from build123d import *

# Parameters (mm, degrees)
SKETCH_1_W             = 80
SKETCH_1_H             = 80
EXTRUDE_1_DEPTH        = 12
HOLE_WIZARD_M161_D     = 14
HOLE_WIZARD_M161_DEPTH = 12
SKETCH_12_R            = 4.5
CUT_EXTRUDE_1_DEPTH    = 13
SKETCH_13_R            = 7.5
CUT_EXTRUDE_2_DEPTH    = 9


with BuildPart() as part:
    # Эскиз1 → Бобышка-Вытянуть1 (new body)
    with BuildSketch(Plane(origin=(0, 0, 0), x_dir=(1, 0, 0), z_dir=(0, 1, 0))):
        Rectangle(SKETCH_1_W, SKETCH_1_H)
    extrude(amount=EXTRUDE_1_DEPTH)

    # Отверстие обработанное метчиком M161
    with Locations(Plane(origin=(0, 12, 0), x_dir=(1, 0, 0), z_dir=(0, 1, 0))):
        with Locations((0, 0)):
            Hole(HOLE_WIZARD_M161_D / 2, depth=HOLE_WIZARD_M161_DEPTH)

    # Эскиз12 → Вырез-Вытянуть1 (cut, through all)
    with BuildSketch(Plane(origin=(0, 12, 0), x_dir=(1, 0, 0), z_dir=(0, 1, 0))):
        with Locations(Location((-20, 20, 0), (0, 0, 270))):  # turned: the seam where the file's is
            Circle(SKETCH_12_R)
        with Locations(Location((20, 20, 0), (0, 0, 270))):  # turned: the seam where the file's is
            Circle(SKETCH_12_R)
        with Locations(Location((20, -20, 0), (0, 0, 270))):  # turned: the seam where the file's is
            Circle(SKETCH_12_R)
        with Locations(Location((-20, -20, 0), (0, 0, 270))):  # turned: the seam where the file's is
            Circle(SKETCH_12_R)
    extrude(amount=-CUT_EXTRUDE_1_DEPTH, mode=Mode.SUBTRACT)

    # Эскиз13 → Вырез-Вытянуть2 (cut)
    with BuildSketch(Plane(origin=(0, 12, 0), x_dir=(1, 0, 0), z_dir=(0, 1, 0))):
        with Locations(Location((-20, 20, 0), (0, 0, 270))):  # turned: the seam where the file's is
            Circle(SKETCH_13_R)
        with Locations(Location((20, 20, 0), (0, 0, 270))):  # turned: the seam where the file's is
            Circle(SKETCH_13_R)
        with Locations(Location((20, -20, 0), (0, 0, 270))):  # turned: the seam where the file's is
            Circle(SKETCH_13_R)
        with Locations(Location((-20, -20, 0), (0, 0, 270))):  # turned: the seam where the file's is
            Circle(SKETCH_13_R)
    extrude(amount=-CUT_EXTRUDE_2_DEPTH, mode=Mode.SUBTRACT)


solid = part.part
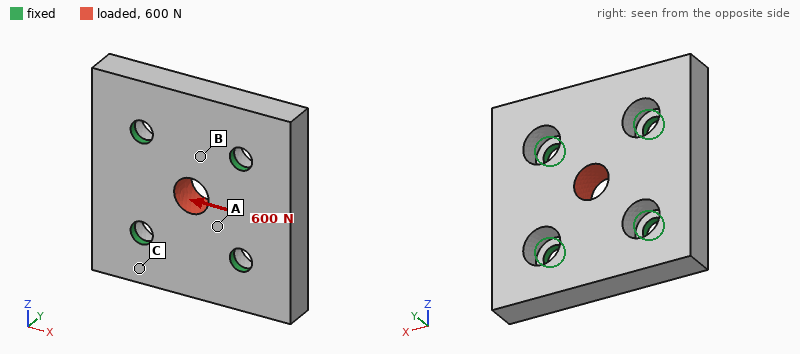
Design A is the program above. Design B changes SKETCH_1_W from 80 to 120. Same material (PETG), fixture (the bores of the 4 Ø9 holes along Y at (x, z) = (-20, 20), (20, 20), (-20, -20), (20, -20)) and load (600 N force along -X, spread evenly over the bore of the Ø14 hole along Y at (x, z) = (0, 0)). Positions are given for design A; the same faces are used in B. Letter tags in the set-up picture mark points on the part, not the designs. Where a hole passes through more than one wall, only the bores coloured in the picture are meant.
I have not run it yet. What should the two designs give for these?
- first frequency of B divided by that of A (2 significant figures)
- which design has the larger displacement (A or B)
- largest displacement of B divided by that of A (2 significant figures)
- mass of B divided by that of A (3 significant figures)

0.39
B
1.4
1.57
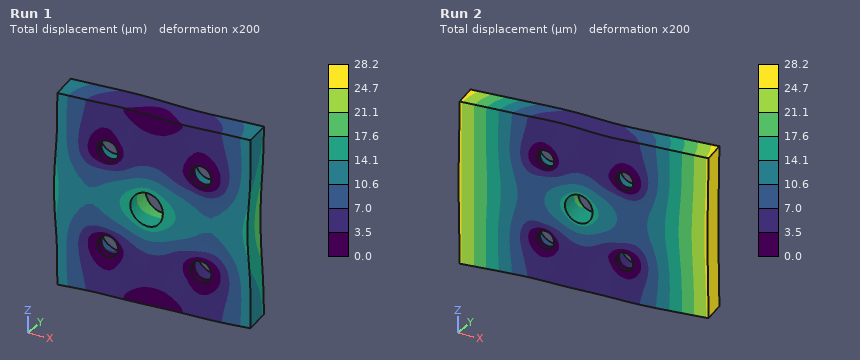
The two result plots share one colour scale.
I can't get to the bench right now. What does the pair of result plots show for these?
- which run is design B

Run 2
